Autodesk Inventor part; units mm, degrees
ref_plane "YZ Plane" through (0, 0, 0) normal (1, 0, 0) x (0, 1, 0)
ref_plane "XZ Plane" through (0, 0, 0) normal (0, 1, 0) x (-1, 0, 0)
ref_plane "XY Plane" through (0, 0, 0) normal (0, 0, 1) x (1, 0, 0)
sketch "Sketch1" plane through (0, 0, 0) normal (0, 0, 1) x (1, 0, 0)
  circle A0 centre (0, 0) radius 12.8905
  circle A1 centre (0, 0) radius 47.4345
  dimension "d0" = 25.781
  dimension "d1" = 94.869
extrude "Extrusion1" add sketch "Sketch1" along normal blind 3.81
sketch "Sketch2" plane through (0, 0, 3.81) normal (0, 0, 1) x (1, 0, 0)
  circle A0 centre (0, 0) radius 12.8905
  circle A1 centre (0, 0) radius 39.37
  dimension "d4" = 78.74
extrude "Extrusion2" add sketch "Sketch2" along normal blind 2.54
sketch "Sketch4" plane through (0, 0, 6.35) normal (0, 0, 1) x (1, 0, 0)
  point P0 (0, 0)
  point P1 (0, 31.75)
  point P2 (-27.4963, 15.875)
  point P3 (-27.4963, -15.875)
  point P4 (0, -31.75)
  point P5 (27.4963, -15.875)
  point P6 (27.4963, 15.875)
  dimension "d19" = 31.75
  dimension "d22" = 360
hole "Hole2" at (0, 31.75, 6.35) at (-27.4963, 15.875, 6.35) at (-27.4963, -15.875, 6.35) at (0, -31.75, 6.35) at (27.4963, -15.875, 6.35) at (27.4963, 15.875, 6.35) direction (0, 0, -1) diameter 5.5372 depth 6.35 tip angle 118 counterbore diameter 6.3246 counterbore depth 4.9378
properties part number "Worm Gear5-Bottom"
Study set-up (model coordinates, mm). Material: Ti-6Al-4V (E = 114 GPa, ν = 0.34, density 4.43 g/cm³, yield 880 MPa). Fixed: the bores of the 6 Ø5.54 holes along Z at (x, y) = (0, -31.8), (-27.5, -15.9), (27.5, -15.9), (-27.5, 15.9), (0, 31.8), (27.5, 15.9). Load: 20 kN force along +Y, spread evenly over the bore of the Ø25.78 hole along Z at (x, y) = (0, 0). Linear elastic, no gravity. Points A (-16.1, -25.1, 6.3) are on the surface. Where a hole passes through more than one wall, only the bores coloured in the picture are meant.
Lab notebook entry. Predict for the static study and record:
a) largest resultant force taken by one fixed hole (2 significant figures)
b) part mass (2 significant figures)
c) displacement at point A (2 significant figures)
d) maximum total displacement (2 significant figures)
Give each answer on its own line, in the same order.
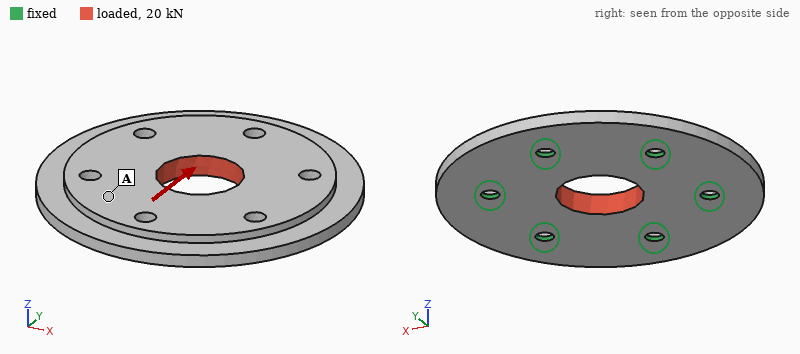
4.1 kN
150 g
9.2 µm
16 µm
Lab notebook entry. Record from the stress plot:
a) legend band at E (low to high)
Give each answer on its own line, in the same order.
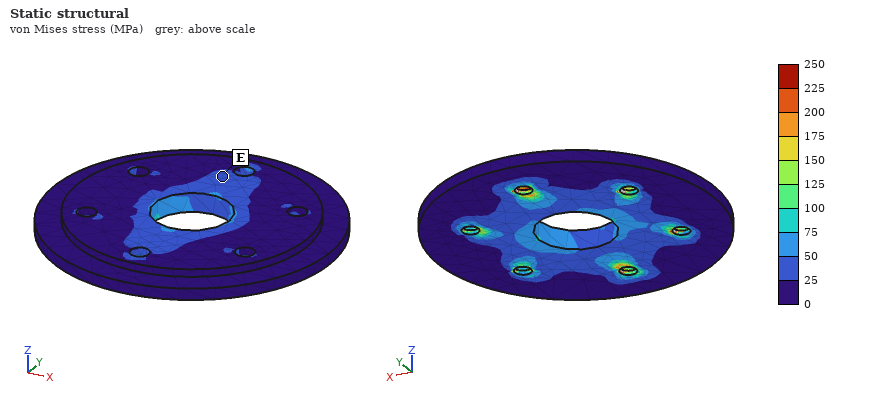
25 to 50 MPa
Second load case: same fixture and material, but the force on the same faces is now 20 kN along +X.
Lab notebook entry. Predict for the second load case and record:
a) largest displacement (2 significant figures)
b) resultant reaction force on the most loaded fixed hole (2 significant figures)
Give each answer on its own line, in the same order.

17 µm
3.8 kN
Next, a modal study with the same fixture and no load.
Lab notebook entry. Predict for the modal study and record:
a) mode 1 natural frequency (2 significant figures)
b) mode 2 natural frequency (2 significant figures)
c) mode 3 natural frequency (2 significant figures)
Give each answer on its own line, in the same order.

9700 Hz
11 kHz
11 kHz
